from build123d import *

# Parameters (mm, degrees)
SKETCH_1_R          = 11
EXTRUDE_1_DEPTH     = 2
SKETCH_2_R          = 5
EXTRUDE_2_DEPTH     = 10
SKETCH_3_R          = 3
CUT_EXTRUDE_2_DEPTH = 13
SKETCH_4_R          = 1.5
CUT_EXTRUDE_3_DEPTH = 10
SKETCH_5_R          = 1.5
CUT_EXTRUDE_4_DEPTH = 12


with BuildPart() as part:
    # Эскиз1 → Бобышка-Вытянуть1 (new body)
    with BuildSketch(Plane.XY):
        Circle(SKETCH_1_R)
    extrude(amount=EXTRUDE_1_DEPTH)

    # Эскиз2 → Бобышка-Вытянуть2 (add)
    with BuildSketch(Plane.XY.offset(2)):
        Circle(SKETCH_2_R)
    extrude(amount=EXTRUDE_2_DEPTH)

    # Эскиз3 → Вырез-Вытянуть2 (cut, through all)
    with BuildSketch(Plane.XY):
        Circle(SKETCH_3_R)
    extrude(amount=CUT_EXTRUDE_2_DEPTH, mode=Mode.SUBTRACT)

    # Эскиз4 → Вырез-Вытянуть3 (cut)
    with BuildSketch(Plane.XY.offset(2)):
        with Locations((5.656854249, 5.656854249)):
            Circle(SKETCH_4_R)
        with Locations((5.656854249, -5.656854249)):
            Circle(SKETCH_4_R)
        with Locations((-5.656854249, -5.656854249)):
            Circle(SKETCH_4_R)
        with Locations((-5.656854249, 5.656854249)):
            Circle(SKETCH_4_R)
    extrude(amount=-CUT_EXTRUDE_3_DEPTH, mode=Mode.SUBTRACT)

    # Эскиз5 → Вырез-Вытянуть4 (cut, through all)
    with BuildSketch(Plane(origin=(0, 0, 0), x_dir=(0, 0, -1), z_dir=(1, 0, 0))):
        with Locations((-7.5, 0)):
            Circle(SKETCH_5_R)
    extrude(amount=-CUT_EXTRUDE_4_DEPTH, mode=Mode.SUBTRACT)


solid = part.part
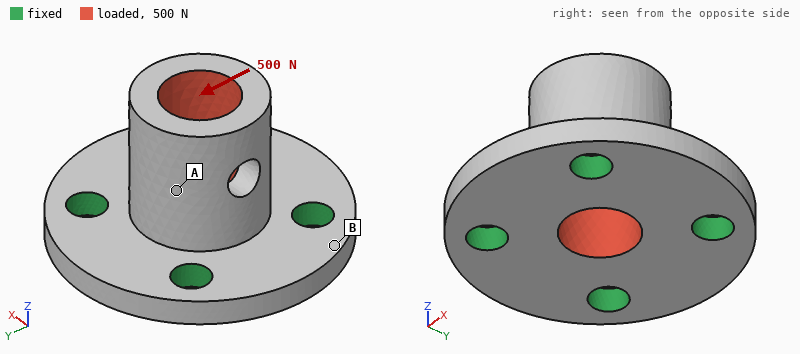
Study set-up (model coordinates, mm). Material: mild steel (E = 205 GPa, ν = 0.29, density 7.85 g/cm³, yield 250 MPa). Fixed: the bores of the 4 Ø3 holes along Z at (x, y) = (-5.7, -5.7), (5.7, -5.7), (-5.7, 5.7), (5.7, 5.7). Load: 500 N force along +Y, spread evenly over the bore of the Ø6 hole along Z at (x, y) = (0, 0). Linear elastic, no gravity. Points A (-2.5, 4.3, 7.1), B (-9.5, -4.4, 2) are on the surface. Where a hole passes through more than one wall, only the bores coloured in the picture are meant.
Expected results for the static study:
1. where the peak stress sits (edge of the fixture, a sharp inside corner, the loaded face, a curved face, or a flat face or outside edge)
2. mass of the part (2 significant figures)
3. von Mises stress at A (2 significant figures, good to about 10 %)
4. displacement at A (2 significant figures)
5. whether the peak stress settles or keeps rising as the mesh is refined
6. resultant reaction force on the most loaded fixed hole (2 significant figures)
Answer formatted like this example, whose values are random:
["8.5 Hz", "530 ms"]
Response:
["edge of the fixture", "8.9 g", "12 MPa", "2.4 µm", "keeps rising", "190 N"]
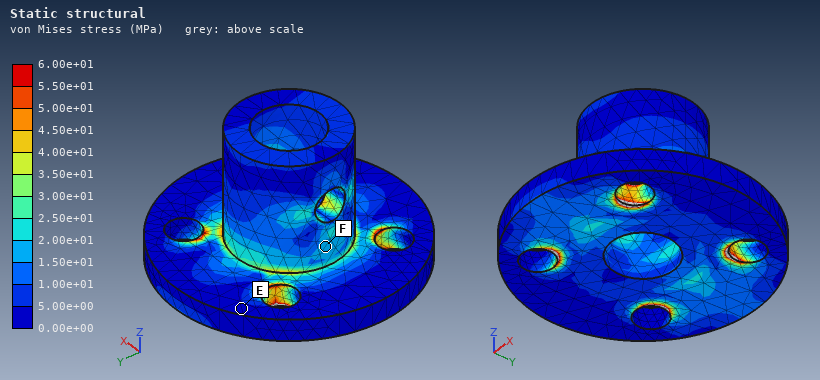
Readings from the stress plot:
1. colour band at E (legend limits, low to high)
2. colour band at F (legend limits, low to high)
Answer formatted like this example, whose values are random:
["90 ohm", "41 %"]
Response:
["0.00e+00 to 5.00e+00 MPa", "1.50e+01 to 2.00e+01 MPa"]
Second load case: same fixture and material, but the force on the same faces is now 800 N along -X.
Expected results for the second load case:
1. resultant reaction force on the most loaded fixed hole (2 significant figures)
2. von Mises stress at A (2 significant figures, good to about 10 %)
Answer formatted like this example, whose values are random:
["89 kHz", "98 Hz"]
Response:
["300 N", "14 MPa"]
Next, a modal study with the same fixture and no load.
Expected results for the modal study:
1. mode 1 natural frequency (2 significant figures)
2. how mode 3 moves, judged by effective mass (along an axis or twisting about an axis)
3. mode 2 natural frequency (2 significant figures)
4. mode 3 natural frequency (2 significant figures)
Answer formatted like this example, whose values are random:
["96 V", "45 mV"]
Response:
["30 kHz", "along Z", "31 kHz", "53 kHz"]
